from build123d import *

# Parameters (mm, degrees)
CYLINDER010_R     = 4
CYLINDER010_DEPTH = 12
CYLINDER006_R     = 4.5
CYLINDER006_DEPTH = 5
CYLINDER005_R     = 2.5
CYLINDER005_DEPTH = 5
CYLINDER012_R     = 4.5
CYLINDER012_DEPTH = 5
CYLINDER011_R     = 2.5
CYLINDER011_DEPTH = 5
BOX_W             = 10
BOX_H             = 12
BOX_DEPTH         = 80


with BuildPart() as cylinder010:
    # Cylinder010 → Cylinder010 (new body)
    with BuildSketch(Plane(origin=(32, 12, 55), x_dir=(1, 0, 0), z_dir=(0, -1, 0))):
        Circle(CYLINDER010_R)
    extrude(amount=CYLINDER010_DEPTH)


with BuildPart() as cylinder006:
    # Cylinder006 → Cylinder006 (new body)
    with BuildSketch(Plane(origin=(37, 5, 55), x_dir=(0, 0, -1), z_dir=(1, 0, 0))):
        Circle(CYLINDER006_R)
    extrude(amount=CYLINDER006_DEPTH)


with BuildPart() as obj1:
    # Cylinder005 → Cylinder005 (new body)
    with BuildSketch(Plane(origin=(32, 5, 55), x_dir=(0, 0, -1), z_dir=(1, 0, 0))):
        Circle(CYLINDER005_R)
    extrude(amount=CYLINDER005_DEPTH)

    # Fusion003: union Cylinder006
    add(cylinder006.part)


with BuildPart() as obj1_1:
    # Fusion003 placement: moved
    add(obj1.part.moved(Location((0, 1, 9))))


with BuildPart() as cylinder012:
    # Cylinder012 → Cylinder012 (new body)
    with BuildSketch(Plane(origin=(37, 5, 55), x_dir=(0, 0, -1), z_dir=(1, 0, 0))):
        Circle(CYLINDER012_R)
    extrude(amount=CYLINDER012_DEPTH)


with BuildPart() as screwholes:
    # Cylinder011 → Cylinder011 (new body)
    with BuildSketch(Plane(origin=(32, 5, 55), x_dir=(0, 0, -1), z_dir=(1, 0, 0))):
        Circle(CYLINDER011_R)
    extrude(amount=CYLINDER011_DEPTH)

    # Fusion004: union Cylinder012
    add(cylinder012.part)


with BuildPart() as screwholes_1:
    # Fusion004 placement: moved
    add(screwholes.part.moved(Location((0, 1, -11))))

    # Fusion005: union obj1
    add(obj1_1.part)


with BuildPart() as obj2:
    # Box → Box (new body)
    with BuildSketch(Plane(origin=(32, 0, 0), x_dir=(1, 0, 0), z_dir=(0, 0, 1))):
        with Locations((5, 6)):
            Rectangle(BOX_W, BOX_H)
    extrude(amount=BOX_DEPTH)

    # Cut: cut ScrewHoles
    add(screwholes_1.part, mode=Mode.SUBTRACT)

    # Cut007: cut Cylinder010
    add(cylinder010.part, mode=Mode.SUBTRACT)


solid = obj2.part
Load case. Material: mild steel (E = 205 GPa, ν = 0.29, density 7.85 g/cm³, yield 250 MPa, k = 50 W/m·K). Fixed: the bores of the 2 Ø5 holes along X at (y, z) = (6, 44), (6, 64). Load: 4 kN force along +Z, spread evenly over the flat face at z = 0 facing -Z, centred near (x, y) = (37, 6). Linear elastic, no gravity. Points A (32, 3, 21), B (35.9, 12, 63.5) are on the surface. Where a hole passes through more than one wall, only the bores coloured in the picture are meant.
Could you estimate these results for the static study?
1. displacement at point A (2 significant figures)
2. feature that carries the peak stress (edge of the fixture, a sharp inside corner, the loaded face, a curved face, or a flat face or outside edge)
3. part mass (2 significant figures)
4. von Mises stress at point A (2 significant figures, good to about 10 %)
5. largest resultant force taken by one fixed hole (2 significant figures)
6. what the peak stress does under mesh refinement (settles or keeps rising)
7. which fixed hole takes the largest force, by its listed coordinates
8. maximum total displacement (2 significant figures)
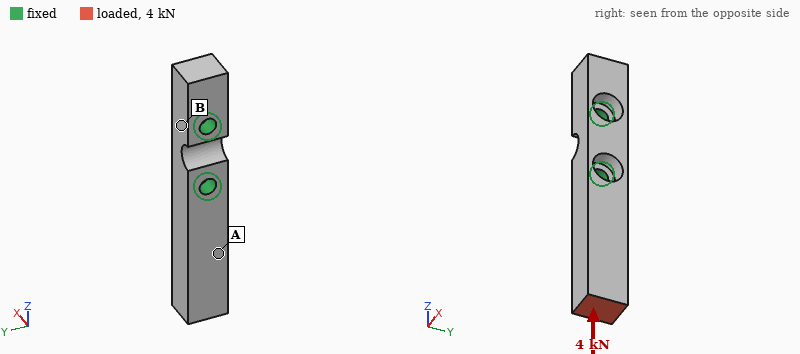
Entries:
12 µm
edge of the fixture
66 g
33 MPa
3.5 kN
keeps rising
(6, 44)
27 µm
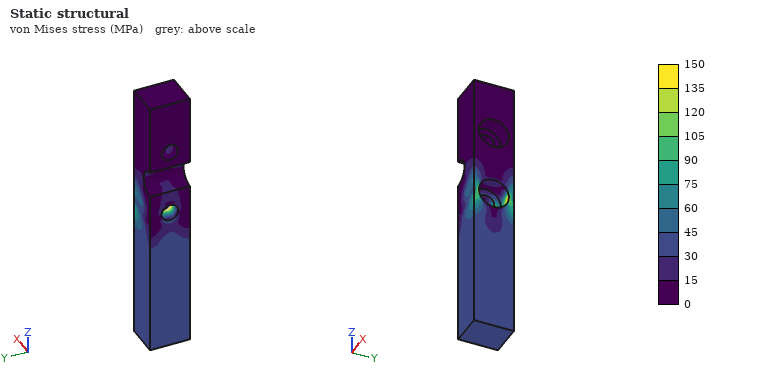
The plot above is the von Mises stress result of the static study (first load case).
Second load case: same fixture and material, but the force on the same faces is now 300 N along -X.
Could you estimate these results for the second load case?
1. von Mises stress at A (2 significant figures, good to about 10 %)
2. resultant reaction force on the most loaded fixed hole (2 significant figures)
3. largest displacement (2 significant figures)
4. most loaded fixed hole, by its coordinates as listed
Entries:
31 MPa
730 N
67 µm
(6, 44)
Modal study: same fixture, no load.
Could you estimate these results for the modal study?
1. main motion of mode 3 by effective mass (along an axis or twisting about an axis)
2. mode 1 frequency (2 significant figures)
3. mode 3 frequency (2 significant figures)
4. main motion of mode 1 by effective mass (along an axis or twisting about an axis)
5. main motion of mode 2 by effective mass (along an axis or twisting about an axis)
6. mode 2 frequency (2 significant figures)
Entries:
twisting about Z
3200 Hz
14 kHz
along X
along Y
4000 Hz
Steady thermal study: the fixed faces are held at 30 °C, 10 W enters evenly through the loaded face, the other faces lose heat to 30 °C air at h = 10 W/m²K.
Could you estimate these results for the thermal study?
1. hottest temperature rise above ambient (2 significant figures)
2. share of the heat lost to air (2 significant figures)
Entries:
73 K
7.5 %
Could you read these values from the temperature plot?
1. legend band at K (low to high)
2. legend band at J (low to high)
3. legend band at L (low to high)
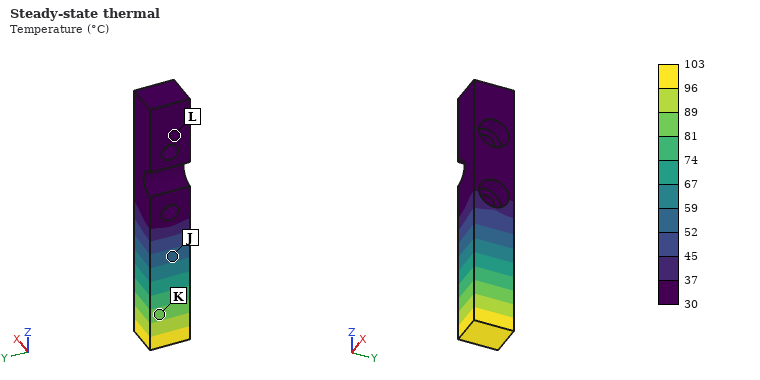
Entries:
81 to 89 °C
52 to 59 °C
30 to 37 °C
